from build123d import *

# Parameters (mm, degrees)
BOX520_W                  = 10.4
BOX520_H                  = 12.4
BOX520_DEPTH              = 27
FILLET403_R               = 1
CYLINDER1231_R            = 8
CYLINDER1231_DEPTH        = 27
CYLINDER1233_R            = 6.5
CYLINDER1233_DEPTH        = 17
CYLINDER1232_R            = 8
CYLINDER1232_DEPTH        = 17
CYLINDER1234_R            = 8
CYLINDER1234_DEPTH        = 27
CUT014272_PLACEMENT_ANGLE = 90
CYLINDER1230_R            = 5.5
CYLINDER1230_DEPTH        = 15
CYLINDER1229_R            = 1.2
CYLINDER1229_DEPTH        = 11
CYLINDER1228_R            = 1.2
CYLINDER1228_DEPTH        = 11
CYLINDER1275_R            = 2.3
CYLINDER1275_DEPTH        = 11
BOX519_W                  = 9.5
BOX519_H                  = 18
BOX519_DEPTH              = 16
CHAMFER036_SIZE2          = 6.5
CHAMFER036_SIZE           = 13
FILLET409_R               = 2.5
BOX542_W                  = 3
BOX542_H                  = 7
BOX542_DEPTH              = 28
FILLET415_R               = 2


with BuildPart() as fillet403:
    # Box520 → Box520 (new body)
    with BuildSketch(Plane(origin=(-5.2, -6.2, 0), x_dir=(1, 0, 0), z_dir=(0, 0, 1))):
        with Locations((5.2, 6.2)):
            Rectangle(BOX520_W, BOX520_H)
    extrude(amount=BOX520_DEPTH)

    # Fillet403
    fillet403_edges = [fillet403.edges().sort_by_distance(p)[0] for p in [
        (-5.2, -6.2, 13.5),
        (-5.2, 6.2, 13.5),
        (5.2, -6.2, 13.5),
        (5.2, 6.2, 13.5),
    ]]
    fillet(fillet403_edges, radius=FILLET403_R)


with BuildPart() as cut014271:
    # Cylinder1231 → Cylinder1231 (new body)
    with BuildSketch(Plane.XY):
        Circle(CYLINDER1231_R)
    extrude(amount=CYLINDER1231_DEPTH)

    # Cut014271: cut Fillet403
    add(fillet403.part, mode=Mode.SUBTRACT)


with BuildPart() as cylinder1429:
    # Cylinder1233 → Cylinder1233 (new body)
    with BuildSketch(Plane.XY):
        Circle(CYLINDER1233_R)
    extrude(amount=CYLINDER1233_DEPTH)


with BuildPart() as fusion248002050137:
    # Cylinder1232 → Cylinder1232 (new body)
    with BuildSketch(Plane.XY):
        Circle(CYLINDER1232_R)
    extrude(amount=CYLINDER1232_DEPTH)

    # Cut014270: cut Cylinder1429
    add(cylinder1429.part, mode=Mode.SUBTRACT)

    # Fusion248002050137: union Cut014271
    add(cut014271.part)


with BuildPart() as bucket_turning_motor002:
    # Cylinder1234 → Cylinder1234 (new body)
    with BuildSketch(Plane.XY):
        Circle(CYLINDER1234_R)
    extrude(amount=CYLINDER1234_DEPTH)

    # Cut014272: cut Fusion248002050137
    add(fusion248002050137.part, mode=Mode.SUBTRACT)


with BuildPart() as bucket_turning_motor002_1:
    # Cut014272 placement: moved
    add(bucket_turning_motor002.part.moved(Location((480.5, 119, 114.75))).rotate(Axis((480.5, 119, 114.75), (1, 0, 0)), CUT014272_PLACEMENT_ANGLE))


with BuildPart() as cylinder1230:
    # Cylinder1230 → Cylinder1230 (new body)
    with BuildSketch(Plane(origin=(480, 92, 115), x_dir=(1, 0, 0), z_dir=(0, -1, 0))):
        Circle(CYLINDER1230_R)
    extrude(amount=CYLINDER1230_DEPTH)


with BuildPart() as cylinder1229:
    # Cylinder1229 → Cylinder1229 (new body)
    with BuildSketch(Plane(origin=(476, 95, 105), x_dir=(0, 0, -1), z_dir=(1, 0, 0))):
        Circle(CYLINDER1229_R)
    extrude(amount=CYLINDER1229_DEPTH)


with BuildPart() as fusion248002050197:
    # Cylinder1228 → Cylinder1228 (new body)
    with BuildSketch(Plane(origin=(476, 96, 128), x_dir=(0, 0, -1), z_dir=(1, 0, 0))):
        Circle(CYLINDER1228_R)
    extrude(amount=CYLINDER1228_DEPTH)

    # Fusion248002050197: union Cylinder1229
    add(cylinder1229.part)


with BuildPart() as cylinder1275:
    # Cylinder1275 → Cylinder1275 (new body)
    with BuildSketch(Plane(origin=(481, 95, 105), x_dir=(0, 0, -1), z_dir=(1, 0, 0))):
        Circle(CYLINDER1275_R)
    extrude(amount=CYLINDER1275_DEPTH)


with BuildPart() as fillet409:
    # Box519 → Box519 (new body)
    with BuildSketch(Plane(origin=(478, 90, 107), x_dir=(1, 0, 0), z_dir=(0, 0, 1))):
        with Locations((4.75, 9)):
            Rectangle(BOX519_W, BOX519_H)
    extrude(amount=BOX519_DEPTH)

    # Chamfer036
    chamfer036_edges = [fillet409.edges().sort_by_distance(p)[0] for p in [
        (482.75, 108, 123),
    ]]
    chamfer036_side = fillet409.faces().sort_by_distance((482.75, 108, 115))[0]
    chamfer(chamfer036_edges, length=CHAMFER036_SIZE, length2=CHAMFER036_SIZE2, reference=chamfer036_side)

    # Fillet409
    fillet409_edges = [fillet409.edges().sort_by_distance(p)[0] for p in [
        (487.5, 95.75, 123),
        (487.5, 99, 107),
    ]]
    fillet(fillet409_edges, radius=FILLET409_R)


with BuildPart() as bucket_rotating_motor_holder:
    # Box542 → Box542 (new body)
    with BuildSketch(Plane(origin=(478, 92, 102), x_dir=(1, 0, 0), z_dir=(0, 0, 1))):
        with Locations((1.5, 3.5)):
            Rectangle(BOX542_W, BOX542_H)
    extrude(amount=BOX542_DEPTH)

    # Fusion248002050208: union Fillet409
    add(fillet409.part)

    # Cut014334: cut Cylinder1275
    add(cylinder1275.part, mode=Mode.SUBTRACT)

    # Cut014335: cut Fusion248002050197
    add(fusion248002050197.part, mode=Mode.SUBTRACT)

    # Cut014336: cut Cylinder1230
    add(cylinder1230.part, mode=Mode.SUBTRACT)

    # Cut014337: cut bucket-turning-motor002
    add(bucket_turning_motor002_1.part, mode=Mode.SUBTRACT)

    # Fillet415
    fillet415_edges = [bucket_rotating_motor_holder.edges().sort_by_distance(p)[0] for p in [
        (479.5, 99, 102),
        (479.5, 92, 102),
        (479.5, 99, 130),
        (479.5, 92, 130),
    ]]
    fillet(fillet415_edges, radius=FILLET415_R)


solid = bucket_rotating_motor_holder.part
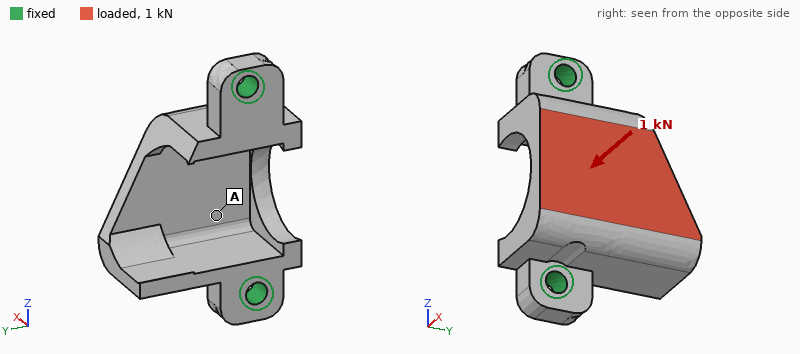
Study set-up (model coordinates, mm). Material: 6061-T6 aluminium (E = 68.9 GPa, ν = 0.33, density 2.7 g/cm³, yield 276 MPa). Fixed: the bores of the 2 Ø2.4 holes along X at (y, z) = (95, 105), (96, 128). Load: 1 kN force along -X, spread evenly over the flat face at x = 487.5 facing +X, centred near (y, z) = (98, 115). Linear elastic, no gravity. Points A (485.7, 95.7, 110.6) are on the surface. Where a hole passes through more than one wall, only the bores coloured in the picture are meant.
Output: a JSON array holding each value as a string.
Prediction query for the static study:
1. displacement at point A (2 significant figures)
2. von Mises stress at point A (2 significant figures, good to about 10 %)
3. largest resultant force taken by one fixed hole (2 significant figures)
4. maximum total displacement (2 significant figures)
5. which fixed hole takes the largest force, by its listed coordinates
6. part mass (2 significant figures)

["27 µm", "27 MPa", "630 N", "80 µm", "(95, 105)", "3.0 g"]
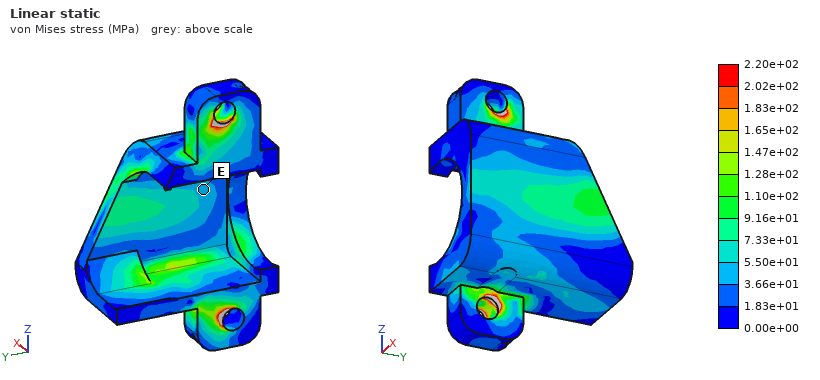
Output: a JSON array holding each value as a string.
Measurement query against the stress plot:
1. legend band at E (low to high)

["3.66e+01 to 5.50e+01 MPa"]
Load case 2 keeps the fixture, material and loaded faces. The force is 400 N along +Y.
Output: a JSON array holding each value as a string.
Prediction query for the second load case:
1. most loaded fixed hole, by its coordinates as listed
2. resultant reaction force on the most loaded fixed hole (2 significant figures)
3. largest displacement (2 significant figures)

["(95, 105)", "240 N", "68 µm"]
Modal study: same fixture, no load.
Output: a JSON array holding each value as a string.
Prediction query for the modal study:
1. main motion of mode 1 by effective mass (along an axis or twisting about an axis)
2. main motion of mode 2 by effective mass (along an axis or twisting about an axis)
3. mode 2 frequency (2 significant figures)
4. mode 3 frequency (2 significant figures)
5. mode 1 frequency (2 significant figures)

["along Y", "along Z", "15 kHz", "24 kHz", "11 kHz"]
